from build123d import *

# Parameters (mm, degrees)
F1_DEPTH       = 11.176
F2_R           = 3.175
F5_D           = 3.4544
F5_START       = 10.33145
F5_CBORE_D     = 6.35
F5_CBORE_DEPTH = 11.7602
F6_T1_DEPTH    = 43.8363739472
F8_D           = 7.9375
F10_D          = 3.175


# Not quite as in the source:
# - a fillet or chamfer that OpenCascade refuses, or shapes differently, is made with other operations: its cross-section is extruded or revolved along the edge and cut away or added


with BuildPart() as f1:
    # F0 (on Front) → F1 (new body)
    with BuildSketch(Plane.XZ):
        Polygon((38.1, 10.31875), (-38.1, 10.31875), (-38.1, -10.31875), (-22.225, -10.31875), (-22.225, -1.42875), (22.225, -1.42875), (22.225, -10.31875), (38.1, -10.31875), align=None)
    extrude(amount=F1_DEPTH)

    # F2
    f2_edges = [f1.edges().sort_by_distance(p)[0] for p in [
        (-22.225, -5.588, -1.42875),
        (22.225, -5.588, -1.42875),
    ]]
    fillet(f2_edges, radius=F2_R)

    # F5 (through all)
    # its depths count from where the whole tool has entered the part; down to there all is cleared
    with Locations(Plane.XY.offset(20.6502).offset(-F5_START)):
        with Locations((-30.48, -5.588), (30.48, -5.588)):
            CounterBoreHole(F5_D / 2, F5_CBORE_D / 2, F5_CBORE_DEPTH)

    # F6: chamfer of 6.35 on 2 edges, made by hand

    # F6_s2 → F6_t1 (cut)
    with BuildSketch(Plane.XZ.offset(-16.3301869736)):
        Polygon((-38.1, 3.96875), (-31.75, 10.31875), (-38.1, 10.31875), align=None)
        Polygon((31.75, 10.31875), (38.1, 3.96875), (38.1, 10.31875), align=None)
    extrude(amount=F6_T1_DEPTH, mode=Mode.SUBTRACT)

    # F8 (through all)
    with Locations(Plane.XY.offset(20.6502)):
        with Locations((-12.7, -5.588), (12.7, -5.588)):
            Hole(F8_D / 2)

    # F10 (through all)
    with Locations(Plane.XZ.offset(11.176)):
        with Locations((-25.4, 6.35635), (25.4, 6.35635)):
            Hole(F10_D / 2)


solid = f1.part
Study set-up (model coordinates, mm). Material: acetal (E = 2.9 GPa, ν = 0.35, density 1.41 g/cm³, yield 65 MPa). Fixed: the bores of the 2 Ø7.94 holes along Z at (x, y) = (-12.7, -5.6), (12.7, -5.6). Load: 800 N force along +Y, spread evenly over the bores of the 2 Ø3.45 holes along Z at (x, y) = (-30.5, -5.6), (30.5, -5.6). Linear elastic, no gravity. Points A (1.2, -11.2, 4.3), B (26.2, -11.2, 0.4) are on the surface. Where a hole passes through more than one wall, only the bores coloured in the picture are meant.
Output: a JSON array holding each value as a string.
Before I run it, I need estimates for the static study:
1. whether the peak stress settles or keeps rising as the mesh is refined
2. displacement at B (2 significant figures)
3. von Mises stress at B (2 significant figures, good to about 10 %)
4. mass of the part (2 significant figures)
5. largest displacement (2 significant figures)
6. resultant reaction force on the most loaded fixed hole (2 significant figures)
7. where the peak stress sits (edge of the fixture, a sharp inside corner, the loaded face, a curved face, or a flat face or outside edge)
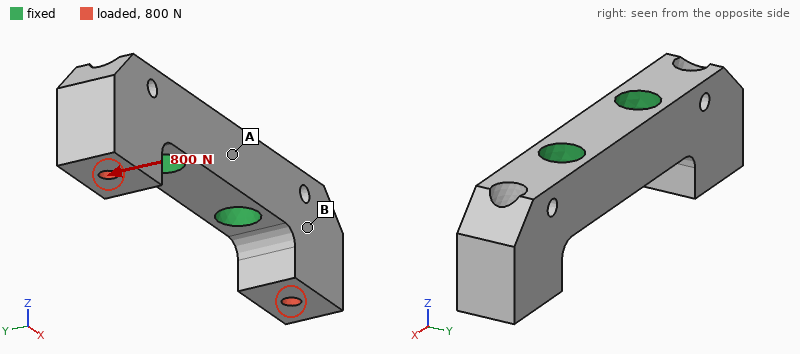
["keeps rising", "0.20 mm", "13 MPa", "15 g", "0.54 mm", "400 N", "edge of the fixture"]
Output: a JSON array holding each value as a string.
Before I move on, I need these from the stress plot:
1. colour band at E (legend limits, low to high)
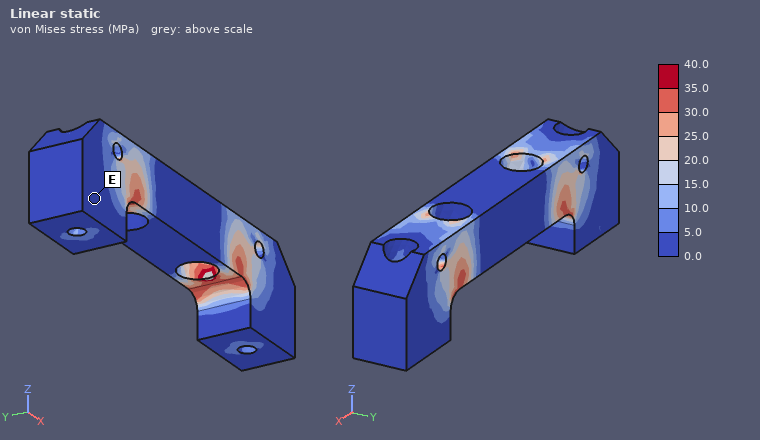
["0.0 to 5.0 MPa"]
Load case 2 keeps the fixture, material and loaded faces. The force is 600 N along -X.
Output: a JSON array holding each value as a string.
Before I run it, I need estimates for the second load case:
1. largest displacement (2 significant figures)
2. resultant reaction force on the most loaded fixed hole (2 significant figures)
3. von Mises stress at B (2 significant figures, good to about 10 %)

["0.20 mm", "300 N", "5.8 MPa"]
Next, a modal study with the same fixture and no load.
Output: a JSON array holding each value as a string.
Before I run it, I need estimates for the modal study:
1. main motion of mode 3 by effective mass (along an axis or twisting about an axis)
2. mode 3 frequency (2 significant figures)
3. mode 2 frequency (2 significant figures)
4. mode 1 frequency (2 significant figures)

["along Z", "3400 Hz", "3100 Hz", "3100 Hz"]
